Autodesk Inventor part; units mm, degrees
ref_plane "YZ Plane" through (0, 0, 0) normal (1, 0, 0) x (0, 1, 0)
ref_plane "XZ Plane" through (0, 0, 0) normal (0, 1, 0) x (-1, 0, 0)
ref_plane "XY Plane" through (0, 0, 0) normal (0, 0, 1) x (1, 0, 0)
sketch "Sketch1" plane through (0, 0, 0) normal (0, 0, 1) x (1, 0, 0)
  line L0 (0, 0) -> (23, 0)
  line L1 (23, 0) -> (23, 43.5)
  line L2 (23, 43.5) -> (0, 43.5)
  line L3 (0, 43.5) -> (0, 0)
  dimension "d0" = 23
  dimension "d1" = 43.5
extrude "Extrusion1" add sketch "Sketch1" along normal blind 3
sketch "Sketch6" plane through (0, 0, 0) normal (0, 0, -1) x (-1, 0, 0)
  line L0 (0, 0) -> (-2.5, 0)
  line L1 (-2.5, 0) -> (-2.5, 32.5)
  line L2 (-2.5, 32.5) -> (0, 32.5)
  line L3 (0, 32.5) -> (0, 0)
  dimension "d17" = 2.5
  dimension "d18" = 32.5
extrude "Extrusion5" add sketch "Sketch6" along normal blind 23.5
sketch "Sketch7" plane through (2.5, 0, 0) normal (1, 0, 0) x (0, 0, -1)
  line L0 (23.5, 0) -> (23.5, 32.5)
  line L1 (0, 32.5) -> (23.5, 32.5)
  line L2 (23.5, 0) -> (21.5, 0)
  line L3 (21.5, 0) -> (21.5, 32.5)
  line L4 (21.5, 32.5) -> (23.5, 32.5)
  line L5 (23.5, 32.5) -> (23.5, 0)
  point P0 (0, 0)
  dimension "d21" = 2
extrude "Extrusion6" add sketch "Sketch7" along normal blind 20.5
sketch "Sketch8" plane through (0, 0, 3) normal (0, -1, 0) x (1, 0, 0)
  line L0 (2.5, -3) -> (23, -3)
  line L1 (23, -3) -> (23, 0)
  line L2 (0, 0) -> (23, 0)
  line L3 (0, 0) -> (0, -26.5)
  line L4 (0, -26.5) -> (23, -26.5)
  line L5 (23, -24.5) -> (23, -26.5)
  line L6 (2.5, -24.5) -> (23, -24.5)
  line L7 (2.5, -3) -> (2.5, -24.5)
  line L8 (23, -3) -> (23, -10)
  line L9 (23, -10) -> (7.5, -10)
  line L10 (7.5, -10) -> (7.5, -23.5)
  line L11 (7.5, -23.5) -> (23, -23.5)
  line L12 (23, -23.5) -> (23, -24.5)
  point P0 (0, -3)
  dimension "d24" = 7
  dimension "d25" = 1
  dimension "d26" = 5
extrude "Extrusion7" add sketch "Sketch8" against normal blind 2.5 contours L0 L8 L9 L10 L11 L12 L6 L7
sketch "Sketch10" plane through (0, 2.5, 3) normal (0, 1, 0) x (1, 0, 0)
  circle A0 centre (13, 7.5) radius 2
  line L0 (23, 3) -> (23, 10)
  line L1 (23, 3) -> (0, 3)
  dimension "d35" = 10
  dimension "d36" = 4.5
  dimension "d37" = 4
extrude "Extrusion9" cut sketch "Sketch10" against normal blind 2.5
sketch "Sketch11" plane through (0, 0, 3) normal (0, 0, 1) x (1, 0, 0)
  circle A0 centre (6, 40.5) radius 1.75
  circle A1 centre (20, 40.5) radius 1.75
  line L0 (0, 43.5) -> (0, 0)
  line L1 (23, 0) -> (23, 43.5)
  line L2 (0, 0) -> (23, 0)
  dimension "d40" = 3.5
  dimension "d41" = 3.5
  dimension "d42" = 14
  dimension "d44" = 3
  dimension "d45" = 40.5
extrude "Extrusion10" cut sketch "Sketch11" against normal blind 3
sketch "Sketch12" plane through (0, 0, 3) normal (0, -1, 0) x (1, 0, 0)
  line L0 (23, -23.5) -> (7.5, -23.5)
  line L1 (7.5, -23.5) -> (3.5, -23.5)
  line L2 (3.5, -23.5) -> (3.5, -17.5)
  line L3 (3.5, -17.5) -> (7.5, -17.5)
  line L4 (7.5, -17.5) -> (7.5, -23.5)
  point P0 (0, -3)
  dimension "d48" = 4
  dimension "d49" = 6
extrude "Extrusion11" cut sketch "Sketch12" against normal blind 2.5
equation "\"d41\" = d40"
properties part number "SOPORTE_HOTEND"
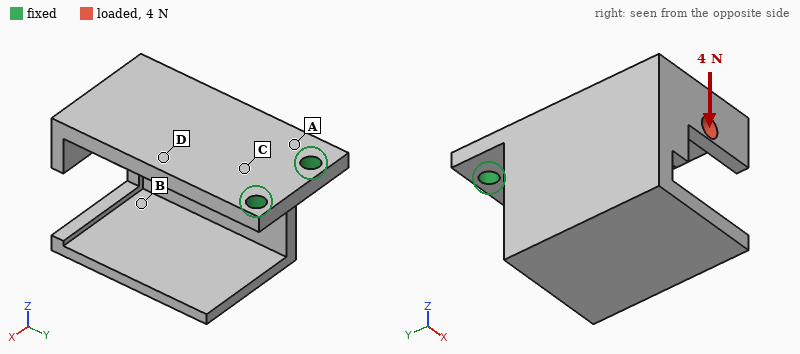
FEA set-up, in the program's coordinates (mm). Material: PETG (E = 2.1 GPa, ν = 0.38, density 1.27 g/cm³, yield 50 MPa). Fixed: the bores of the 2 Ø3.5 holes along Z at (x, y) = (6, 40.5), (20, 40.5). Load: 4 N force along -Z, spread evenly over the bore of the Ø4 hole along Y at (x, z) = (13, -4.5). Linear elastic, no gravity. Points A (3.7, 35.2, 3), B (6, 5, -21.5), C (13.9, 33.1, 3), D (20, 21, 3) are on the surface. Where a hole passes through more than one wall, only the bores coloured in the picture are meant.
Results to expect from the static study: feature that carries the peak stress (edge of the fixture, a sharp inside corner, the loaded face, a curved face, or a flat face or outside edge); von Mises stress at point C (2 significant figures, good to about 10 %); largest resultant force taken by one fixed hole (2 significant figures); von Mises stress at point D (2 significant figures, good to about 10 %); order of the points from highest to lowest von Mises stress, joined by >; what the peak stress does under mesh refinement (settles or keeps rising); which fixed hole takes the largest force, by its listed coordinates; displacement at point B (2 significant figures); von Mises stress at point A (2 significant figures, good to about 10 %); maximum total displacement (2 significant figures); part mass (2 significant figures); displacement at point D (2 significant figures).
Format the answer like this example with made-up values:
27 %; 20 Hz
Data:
edge of the fixture; 2.9 MPa; 2.7 N; 1.2 MPa; A > C > D > B; keeps rising; (6, 40.5); 0.57 mm; 4.4 MPa; 0.65 mm; 8.5 g; 0.18 mm
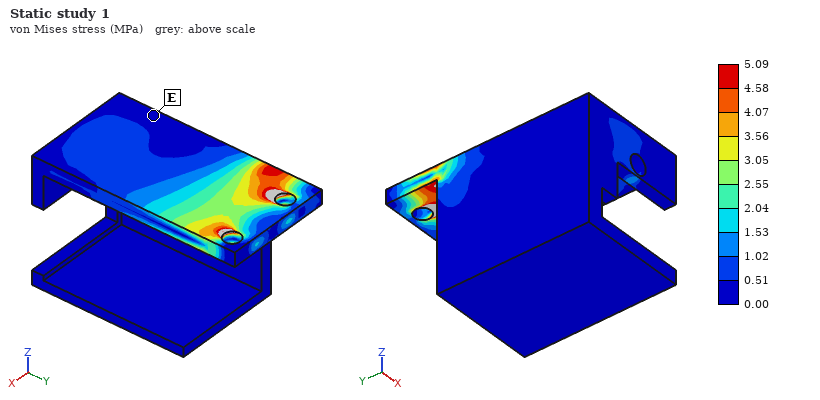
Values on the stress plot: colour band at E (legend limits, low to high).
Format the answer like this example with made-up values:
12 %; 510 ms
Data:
0.00 to 0.51 MPa
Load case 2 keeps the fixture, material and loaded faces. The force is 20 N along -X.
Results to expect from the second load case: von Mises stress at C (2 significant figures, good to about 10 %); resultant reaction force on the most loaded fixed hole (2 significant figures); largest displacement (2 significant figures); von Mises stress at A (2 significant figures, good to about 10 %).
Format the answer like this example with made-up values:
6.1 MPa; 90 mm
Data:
0.98 MPa; 51 N; 0.62 mm; 3.7 MPa
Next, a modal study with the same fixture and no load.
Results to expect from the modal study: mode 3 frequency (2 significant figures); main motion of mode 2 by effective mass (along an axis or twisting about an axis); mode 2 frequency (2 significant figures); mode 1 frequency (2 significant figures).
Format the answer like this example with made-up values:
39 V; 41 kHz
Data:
670 Hz; along X; 300 Hz; 200 Hz
